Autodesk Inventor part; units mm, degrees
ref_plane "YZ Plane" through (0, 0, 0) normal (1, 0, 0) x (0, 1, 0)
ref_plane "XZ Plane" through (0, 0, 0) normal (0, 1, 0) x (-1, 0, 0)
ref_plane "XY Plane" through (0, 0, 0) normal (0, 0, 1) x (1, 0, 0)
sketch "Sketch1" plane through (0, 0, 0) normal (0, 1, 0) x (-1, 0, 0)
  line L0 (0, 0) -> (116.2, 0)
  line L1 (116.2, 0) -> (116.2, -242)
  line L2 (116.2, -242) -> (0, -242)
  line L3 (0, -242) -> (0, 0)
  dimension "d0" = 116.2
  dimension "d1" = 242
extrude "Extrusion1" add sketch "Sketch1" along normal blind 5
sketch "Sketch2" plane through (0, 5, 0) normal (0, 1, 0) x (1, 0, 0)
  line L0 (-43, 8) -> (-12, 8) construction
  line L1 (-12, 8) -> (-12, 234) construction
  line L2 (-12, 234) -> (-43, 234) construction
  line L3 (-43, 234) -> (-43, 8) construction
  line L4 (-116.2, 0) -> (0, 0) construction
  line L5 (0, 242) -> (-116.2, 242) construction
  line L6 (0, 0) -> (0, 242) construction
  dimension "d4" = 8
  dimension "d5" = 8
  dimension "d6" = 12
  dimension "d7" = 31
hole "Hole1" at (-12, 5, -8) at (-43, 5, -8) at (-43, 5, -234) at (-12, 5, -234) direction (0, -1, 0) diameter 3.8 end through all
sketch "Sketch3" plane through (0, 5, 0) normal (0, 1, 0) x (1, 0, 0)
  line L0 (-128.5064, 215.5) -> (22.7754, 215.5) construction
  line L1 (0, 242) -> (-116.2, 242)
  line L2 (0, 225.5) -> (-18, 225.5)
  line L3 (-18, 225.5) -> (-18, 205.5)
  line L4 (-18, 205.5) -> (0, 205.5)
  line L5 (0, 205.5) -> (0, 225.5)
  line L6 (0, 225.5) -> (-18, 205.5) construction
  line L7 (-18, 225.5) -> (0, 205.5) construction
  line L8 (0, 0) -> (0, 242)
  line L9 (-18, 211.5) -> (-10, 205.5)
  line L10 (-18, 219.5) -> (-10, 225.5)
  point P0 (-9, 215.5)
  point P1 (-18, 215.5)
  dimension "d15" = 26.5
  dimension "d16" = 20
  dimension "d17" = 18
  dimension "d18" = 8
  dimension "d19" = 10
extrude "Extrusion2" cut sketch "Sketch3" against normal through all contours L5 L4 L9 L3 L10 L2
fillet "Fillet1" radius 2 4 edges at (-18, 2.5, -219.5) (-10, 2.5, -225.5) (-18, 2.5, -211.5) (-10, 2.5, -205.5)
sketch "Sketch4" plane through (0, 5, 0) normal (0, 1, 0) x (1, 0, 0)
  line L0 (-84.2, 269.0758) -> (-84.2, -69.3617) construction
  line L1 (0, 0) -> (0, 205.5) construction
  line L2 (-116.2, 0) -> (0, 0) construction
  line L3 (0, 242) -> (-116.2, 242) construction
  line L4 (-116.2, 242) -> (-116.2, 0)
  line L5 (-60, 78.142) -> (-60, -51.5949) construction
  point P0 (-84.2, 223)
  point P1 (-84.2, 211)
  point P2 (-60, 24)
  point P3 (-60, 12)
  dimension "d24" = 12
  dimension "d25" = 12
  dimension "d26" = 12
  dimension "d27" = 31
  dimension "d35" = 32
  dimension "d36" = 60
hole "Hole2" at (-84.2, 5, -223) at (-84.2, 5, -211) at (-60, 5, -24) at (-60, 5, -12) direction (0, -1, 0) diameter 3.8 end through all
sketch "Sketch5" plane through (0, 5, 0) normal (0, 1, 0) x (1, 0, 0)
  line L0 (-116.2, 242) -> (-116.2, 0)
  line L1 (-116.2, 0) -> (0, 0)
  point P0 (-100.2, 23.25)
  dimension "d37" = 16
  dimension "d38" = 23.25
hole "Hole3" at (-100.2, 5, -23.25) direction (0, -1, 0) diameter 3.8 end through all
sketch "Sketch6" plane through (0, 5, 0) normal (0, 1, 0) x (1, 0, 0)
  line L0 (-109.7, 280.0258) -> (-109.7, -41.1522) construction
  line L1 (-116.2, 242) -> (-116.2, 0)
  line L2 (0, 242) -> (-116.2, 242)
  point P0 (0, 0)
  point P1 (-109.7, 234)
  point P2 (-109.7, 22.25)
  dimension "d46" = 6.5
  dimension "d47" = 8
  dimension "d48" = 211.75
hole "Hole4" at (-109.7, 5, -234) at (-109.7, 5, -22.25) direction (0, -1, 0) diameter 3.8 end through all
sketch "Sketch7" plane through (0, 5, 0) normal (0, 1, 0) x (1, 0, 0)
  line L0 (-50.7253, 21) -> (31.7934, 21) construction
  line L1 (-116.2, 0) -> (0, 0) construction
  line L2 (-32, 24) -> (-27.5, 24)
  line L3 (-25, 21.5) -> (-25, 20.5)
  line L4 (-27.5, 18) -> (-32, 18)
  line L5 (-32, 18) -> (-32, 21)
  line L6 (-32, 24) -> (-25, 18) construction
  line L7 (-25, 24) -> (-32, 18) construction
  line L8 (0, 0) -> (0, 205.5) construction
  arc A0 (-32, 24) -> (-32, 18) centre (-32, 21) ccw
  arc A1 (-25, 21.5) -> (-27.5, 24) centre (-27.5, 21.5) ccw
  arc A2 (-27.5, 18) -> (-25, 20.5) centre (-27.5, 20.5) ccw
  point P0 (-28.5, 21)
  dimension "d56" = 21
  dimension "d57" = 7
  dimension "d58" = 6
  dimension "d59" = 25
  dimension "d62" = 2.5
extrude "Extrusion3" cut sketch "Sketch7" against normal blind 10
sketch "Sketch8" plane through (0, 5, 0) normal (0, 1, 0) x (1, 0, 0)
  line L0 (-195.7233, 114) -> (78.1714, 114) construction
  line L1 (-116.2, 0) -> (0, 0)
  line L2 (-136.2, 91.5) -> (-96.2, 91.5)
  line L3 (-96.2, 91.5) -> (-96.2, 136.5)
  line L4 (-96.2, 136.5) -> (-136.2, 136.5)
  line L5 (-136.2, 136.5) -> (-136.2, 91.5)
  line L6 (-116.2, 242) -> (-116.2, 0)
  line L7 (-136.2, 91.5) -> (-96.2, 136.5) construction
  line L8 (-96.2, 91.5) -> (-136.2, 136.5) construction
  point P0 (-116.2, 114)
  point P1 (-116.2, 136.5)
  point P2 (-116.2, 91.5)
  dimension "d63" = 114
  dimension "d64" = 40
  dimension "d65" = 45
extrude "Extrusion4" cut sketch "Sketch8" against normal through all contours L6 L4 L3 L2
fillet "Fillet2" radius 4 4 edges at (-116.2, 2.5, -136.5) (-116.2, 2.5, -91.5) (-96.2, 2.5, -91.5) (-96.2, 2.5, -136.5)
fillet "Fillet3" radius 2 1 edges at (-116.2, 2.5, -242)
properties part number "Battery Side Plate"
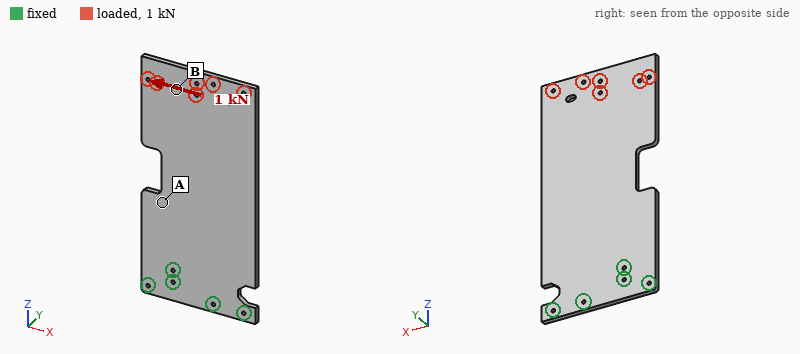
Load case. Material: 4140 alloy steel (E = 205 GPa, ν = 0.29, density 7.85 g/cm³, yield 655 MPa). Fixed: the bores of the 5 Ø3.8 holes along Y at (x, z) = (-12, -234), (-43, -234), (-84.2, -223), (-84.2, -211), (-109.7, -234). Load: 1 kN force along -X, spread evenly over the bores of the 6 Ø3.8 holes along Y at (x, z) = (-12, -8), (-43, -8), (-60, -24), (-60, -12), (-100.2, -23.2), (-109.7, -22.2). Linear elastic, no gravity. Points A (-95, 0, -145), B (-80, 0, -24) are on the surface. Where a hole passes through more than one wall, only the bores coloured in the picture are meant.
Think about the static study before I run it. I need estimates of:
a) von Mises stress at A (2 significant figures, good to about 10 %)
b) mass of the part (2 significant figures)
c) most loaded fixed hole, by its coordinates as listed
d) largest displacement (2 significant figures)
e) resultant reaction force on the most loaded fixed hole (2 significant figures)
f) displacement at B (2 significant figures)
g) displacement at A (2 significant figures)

14 MPa
1.0 kg
(-43, -234)
53 µm
1.8 kN
44 µm
12 µm
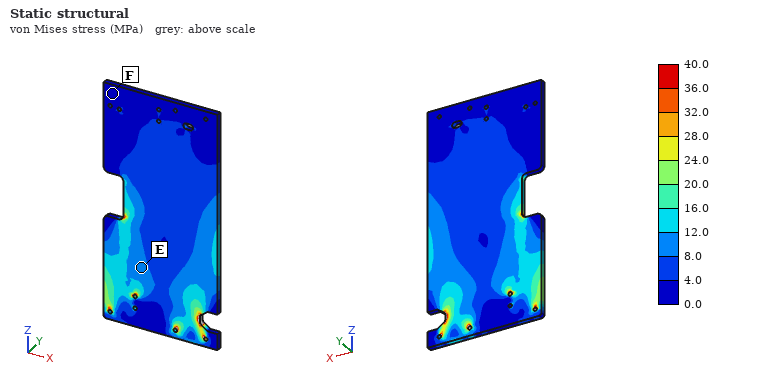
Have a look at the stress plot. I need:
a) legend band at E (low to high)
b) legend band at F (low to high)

8.0 to 12.0 MPa
0.0 to 4.0 MPa
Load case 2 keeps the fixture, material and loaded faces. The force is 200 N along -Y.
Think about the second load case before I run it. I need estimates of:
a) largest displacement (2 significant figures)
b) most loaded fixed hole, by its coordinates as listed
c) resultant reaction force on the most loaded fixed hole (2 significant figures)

2.8 mm
(-84.2, -211)
1.5 kN
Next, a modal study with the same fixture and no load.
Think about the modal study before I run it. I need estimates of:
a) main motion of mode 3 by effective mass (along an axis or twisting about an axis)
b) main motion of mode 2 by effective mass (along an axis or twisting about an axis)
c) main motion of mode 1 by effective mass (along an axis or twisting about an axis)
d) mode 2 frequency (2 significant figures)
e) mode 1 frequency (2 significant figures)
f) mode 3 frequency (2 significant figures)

along Y
twisting about Z
along Y
320 Hz
83 Hz
520 Hz
